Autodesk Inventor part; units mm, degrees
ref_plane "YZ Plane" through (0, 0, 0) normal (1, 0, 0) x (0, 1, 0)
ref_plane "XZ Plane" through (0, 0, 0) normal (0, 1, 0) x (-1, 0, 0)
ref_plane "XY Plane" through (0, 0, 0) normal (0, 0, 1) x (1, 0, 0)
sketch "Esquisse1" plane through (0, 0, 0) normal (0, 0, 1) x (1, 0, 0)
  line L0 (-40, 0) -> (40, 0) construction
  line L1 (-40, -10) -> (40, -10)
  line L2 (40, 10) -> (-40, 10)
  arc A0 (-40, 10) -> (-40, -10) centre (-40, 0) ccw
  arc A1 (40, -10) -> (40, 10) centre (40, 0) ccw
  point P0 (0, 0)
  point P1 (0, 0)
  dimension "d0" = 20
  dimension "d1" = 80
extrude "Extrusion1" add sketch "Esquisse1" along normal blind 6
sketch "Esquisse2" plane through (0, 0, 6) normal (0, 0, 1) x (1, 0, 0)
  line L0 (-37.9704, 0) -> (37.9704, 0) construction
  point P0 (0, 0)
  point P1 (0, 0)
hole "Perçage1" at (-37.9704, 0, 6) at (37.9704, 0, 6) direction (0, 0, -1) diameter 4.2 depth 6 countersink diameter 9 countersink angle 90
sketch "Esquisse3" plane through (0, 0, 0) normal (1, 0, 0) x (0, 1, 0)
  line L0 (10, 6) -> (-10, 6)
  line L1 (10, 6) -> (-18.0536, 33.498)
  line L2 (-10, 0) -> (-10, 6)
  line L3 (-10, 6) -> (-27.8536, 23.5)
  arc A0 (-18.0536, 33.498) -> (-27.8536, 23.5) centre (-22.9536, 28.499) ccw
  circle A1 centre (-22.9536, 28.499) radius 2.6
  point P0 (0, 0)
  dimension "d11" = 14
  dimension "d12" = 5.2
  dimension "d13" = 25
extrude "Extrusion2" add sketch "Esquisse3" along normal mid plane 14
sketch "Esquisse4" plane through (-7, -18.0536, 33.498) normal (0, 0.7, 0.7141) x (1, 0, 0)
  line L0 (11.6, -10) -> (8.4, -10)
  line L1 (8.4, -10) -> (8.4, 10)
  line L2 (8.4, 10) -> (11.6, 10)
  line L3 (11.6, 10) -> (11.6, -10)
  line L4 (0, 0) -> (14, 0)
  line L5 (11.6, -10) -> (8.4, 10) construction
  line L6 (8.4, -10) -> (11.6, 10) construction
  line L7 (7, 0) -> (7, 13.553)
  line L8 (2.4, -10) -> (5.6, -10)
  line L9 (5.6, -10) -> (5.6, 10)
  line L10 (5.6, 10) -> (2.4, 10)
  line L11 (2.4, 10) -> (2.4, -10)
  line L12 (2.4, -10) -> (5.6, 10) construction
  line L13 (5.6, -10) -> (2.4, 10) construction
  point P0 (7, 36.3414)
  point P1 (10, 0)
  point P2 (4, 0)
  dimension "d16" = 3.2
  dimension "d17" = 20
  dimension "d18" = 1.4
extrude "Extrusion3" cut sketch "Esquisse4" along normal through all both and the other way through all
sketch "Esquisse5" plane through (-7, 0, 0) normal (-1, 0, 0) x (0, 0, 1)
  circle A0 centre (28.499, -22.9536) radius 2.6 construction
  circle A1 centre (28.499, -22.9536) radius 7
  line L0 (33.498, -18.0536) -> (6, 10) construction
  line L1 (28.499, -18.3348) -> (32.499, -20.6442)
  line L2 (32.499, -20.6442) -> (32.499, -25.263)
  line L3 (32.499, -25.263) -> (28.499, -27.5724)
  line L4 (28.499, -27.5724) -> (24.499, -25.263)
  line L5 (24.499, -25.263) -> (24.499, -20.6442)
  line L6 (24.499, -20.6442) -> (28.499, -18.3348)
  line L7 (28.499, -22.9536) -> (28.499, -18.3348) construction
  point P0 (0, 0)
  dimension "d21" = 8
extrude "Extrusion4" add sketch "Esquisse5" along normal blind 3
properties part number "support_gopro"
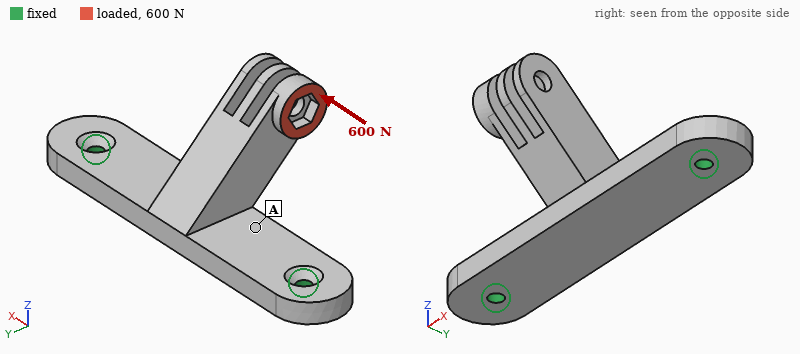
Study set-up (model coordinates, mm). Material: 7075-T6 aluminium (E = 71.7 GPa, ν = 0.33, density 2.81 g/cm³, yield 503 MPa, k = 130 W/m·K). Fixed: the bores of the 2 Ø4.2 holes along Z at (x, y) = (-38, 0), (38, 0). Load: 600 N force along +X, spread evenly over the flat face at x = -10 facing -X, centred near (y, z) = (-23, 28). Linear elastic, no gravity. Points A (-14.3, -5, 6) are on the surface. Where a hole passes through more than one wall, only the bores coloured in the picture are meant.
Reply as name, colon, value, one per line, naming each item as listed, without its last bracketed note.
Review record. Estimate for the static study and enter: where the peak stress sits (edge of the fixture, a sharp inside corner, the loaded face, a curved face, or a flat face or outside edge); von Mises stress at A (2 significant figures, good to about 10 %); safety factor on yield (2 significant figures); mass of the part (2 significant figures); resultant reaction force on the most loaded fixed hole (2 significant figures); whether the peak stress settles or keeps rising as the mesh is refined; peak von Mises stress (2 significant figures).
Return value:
where the peak stress sits: a flat face or outside edge
von Mises stress at A: 39 MPa
safety factor on yield: 1.3
mass of the part: 49 g
resultant reaction force on the most loaded fixed hole: 450 N
whether the peak stress settles or keeps rising as the mesh is refined: settles
peak von Mises stress: 380 MPa
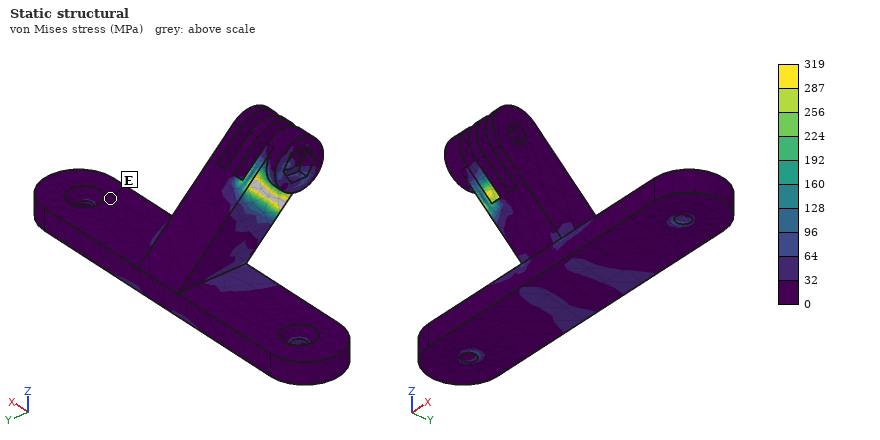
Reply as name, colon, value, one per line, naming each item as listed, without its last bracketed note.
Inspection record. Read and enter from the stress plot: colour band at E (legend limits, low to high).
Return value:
colour band at E: 0 to 32 MPa
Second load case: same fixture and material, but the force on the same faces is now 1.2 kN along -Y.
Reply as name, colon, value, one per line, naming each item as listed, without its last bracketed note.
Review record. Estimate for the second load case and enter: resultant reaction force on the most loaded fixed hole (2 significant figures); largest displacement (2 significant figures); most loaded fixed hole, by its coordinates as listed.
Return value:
resultant reaction force on the most loaded fixed hole: 770 N
largest displacement: 0.93 mm
most loaded fixed hole, by its coordinates as listed: (-38, 0)
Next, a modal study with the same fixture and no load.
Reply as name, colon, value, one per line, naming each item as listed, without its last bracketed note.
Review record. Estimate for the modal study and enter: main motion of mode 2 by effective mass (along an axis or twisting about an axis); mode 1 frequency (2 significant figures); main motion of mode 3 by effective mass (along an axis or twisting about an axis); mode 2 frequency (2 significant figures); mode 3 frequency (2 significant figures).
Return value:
main motion of mode 2 by effective mass: along Z
mode 1 frequency: 2100 Hz
main motion of mode 3 by effective mass: along X
mode 2 frequency: 3500 Hz
mode 3 frequency: 4200 Hz
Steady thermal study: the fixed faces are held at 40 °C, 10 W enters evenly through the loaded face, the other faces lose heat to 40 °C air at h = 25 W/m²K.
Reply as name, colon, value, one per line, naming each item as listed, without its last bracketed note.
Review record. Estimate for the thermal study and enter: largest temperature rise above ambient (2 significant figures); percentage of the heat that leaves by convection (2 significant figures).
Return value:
largest temperature rise above ambient: 44 K
percentage of the heat that leaves by convection: 19 %
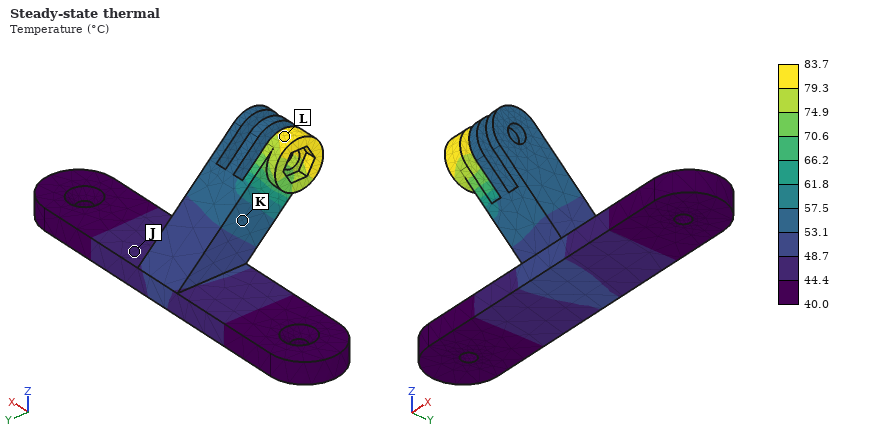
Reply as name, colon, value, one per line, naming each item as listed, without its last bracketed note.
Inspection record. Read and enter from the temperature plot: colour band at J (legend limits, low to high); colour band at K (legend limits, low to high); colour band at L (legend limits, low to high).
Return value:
colour band at J: 44.4 to 48.7 °C
colour band at K: 53.1 to 57.5 °C
colour band at L: 79.3 to 83.7 °C
